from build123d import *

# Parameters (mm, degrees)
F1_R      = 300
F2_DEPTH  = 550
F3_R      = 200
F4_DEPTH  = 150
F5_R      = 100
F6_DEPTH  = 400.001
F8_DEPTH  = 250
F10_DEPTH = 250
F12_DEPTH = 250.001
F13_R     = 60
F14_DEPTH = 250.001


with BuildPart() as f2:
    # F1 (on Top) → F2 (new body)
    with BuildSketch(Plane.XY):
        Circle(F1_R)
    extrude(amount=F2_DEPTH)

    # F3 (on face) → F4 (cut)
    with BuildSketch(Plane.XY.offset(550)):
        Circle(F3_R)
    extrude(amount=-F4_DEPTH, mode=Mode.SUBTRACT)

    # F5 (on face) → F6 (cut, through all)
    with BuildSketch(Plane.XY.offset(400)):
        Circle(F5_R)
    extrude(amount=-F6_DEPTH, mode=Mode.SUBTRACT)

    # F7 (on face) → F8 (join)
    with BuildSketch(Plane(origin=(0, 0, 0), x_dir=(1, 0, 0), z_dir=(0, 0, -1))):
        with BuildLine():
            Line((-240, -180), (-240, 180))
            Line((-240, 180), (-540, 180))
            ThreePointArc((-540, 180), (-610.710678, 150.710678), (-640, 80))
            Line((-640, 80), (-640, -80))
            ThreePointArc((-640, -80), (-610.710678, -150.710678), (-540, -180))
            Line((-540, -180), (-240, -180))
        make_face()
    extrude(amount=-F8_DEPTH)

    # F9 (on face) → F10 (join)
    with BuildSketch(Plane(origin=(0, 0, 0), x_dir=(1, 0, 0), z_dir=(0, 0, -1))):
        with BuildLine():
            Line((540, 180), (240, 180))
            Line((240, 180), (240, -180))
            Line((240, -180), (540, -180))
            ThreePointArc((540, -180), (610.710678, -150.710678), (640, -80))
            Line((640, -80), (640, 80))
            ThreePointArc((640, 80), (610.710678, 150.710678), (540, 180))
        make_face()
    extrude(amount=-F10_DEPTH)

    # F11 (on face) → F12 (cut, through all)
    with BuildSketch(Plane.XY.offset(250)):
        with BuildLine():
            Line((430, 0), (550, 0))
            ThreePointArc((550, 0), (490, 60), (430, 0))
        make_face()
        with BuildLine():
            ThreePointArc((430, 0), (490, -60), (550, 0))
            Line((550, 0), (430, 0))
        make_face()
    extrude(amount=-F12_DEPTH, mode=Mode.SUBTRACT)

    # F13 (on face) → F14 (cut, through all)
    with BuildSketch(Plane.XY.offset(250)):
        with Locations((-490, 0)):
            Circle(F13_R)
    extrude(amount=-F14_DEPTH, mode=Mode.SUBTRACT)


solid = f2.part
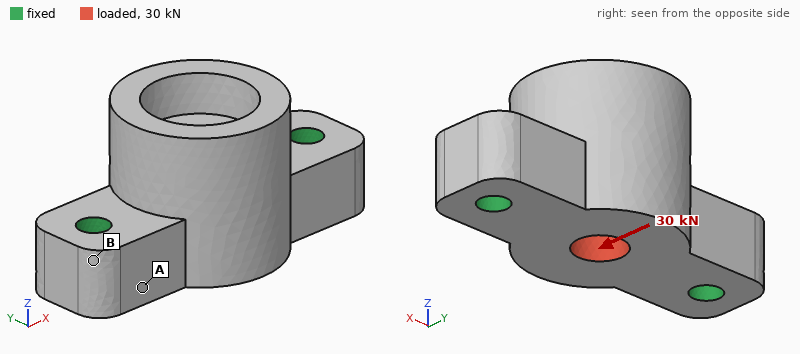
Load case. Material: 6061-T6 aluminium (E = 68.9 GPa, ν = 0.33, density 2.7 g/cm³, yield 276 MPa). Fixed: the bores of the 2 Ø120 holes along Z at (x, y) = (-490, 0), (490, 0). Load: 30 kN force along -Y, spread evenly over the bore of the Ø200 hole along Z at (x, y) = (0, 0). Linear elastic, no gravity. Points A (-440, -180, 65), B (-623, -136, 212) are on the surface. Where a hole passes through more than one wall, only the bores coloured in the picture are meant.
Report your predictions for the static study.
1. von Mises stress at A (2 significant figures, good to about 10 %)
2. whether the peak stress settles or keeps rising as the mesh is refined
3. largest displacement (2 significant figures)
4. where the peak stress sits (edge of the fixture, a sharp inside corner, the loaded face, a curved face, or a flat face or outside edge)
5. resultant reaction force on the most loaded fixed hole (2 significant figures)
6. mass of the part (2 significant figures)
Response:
0.24 MPa
keeps rising
8.3 µm
edge of the fixture
15 kN
490 kg
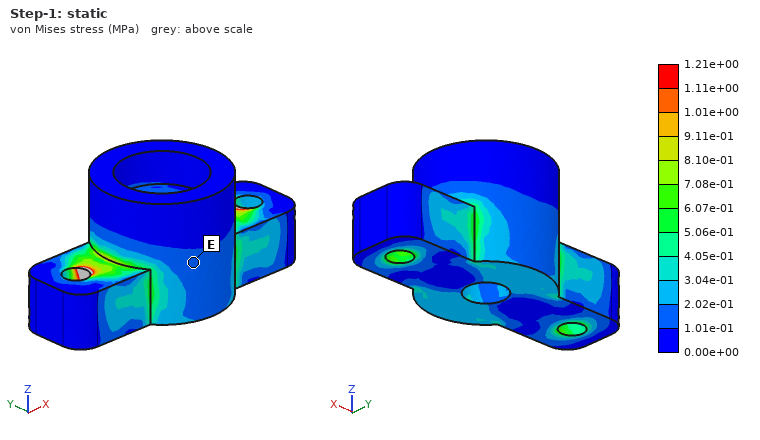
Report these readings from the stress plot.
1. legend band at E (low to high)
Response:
1.01e-01 to 2.02e-01 MPa
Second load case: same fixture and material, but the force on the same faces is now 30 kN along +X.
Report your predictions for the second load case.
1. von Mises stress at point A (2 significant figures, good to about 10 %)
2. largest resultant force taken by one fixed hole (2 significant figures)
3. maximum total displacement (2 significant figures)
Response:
0.066 MPa
15 kN
1.4 µm
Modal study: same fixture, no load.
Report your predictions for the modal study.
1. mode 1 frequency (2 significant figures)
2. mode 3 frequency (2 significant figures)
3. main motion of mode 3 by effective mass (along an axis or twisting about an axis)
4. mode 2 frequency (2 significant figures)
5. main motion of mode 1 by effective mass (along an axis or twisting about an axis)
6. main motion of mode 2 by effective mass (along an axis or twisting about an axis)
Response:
460 Hz
1000 Hz
along Y
790 Hz
along Y
along Z
